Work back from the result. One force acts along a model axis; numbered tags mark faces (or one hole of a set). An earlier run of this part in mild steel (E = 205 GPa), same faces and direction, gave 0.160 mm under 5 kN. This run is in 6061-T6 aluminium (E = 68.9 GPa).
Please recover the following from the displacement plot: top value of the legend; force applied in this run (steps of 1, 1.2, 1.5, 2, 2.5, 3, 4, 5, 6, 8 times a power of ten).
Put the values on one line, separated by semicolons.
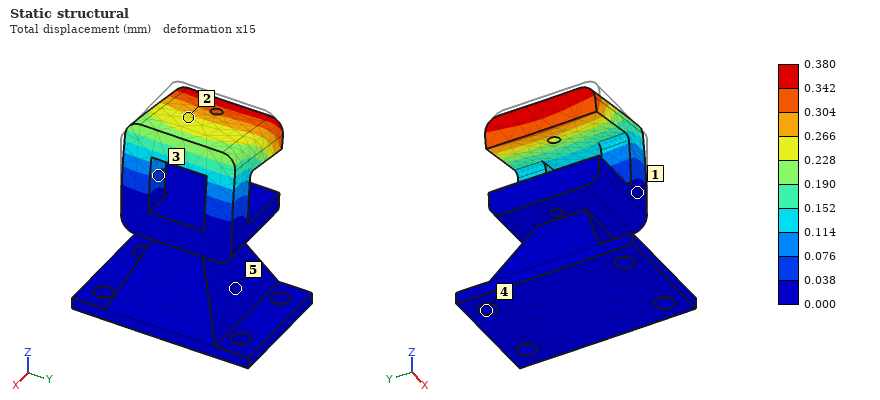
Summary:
0.380 mm; 4 kN
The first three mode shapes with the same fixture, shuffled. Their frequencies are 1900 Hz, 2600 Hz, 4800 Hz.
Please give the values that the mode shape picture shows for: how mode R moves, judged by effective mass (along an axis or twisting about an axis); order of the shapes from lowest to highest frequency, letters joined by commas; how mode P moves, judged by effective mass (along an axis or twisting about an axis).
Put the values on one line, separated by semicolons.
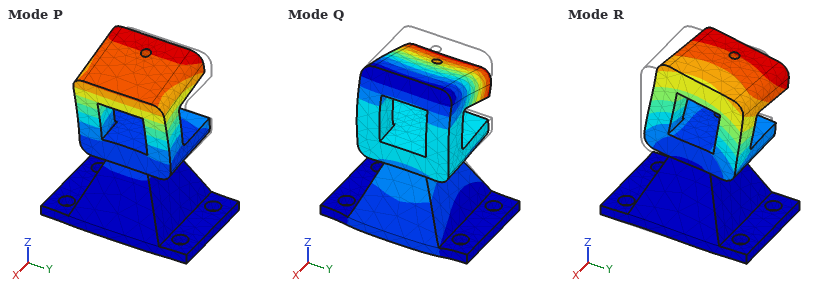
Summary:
along Y; P, R, Q; along X
